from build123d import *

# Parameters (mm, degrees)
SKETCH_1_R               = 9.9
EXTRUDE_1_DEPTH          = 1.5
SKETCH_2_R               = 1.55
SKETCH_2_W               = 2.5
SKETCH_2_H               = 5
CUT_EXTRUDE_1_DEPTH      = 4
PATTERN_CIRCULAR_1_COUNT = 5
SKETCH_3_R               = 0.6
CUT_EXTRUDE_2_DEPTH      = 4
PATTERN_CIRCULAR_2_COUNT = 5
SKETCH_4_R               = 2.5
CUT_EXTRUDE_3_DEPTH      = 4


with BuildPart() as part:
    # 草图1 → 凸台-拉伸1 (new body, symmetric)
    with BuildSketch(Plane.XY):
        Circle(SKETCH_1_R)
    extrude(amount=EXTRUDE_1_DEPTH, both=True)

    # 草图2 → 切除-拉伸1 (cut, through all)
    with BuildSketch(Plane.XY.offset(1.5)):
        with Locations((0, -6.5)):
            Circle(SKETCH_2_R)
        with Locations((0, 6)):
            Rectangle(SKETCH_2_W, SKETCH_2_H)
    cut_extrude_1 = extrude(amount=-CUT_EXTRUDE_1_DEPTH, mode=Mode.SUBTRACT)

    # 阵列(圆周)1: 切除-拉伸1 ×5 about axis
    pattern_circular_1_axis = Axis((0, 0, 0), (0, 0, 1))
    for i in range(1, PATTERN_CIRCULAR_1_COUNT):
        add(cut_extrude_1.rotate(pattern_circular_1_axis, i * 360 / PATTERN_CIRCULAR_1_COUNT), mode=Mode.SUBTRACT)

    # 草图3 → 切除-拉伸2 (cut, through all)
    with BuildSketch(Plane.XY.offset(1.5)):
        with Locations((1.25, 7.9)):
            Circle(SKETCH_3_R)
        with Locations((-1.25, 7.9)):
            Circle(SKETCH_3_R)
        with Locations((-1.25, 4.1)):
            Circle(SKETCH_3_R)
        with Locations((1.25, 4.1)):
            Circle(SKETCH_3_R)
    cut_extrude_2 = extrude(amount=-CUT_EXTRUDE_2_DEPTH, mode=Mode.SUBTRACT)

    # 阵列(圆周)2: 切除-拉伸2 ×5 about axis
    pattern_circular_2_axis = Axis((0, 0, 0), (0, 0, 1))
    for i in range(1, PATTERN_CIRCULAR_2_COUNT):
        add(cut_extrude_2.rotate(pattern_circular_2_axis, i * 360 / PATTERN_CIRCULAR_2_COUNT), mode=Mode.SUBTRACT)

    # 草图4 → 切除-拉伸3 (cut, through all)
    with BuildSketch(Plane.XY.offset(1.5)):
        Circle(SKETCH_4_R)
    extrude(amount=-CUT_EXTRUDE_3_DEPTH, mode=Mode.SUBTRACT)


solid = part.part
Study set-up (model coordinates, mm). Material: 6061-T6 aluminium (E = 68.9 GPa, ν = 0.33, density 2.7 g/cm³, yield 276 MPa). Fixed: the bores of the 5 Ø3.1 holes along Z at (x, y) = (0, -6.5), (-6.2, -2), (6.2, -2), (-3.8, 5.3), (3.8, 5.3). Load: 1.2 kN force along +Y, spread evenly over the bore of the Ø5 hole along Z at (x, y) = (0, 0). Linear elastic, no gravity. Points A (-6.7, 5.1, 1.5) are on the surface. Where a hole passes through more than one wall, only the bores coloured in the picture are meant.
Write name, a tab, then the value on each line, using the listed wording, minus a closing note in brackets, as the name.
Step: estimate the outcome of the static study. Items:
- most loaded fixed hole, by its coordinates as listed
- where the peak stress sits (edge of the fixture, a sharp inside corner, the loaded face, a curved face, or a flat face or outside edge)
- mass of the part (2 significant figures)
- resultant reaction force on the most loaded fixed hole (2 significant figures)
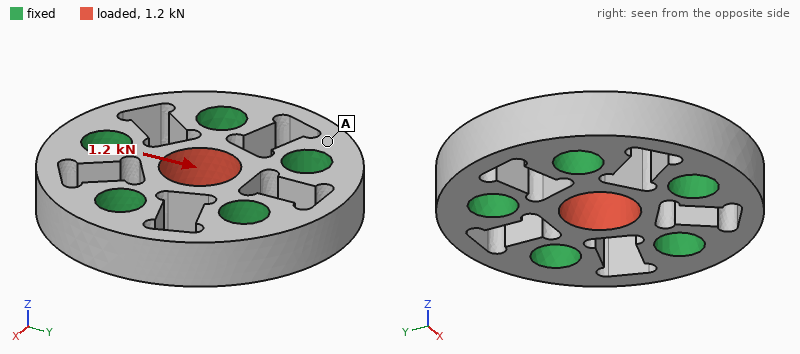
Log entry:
most loaded fixed hole, by its coordinates as listed	(0, -6.5)
where the peak stress sits	a curved face
mass of the part	1.4 g
resultant reaction force on the most loaded fixed hole	360 N
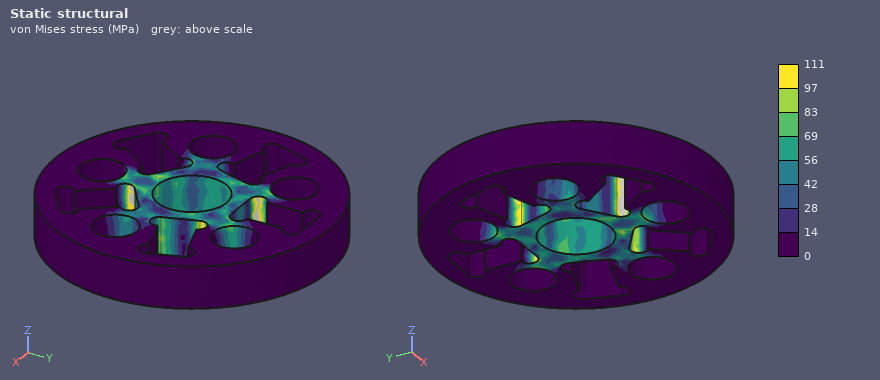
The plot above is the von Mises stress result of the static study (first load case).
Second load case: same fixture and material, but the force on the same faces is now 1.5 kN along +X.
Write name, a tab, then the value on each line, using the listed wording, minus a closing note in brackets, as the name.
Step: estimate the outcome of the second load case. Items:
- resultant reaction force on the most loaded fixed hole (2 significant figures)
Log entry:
resultant reaction force on the most loaded fixed hole	430 N
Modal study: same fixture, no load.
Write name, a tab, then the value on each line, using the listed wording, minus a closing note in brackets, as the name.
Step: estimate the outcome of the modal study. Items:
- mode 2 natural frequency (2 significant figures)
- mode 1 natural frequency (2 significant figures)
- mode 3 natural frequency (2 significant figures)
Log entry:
mode 2 natural frequency	130 kHz
mode 1 natural frequency	130 kHz
mode 3 natural frequency	130 kHz
